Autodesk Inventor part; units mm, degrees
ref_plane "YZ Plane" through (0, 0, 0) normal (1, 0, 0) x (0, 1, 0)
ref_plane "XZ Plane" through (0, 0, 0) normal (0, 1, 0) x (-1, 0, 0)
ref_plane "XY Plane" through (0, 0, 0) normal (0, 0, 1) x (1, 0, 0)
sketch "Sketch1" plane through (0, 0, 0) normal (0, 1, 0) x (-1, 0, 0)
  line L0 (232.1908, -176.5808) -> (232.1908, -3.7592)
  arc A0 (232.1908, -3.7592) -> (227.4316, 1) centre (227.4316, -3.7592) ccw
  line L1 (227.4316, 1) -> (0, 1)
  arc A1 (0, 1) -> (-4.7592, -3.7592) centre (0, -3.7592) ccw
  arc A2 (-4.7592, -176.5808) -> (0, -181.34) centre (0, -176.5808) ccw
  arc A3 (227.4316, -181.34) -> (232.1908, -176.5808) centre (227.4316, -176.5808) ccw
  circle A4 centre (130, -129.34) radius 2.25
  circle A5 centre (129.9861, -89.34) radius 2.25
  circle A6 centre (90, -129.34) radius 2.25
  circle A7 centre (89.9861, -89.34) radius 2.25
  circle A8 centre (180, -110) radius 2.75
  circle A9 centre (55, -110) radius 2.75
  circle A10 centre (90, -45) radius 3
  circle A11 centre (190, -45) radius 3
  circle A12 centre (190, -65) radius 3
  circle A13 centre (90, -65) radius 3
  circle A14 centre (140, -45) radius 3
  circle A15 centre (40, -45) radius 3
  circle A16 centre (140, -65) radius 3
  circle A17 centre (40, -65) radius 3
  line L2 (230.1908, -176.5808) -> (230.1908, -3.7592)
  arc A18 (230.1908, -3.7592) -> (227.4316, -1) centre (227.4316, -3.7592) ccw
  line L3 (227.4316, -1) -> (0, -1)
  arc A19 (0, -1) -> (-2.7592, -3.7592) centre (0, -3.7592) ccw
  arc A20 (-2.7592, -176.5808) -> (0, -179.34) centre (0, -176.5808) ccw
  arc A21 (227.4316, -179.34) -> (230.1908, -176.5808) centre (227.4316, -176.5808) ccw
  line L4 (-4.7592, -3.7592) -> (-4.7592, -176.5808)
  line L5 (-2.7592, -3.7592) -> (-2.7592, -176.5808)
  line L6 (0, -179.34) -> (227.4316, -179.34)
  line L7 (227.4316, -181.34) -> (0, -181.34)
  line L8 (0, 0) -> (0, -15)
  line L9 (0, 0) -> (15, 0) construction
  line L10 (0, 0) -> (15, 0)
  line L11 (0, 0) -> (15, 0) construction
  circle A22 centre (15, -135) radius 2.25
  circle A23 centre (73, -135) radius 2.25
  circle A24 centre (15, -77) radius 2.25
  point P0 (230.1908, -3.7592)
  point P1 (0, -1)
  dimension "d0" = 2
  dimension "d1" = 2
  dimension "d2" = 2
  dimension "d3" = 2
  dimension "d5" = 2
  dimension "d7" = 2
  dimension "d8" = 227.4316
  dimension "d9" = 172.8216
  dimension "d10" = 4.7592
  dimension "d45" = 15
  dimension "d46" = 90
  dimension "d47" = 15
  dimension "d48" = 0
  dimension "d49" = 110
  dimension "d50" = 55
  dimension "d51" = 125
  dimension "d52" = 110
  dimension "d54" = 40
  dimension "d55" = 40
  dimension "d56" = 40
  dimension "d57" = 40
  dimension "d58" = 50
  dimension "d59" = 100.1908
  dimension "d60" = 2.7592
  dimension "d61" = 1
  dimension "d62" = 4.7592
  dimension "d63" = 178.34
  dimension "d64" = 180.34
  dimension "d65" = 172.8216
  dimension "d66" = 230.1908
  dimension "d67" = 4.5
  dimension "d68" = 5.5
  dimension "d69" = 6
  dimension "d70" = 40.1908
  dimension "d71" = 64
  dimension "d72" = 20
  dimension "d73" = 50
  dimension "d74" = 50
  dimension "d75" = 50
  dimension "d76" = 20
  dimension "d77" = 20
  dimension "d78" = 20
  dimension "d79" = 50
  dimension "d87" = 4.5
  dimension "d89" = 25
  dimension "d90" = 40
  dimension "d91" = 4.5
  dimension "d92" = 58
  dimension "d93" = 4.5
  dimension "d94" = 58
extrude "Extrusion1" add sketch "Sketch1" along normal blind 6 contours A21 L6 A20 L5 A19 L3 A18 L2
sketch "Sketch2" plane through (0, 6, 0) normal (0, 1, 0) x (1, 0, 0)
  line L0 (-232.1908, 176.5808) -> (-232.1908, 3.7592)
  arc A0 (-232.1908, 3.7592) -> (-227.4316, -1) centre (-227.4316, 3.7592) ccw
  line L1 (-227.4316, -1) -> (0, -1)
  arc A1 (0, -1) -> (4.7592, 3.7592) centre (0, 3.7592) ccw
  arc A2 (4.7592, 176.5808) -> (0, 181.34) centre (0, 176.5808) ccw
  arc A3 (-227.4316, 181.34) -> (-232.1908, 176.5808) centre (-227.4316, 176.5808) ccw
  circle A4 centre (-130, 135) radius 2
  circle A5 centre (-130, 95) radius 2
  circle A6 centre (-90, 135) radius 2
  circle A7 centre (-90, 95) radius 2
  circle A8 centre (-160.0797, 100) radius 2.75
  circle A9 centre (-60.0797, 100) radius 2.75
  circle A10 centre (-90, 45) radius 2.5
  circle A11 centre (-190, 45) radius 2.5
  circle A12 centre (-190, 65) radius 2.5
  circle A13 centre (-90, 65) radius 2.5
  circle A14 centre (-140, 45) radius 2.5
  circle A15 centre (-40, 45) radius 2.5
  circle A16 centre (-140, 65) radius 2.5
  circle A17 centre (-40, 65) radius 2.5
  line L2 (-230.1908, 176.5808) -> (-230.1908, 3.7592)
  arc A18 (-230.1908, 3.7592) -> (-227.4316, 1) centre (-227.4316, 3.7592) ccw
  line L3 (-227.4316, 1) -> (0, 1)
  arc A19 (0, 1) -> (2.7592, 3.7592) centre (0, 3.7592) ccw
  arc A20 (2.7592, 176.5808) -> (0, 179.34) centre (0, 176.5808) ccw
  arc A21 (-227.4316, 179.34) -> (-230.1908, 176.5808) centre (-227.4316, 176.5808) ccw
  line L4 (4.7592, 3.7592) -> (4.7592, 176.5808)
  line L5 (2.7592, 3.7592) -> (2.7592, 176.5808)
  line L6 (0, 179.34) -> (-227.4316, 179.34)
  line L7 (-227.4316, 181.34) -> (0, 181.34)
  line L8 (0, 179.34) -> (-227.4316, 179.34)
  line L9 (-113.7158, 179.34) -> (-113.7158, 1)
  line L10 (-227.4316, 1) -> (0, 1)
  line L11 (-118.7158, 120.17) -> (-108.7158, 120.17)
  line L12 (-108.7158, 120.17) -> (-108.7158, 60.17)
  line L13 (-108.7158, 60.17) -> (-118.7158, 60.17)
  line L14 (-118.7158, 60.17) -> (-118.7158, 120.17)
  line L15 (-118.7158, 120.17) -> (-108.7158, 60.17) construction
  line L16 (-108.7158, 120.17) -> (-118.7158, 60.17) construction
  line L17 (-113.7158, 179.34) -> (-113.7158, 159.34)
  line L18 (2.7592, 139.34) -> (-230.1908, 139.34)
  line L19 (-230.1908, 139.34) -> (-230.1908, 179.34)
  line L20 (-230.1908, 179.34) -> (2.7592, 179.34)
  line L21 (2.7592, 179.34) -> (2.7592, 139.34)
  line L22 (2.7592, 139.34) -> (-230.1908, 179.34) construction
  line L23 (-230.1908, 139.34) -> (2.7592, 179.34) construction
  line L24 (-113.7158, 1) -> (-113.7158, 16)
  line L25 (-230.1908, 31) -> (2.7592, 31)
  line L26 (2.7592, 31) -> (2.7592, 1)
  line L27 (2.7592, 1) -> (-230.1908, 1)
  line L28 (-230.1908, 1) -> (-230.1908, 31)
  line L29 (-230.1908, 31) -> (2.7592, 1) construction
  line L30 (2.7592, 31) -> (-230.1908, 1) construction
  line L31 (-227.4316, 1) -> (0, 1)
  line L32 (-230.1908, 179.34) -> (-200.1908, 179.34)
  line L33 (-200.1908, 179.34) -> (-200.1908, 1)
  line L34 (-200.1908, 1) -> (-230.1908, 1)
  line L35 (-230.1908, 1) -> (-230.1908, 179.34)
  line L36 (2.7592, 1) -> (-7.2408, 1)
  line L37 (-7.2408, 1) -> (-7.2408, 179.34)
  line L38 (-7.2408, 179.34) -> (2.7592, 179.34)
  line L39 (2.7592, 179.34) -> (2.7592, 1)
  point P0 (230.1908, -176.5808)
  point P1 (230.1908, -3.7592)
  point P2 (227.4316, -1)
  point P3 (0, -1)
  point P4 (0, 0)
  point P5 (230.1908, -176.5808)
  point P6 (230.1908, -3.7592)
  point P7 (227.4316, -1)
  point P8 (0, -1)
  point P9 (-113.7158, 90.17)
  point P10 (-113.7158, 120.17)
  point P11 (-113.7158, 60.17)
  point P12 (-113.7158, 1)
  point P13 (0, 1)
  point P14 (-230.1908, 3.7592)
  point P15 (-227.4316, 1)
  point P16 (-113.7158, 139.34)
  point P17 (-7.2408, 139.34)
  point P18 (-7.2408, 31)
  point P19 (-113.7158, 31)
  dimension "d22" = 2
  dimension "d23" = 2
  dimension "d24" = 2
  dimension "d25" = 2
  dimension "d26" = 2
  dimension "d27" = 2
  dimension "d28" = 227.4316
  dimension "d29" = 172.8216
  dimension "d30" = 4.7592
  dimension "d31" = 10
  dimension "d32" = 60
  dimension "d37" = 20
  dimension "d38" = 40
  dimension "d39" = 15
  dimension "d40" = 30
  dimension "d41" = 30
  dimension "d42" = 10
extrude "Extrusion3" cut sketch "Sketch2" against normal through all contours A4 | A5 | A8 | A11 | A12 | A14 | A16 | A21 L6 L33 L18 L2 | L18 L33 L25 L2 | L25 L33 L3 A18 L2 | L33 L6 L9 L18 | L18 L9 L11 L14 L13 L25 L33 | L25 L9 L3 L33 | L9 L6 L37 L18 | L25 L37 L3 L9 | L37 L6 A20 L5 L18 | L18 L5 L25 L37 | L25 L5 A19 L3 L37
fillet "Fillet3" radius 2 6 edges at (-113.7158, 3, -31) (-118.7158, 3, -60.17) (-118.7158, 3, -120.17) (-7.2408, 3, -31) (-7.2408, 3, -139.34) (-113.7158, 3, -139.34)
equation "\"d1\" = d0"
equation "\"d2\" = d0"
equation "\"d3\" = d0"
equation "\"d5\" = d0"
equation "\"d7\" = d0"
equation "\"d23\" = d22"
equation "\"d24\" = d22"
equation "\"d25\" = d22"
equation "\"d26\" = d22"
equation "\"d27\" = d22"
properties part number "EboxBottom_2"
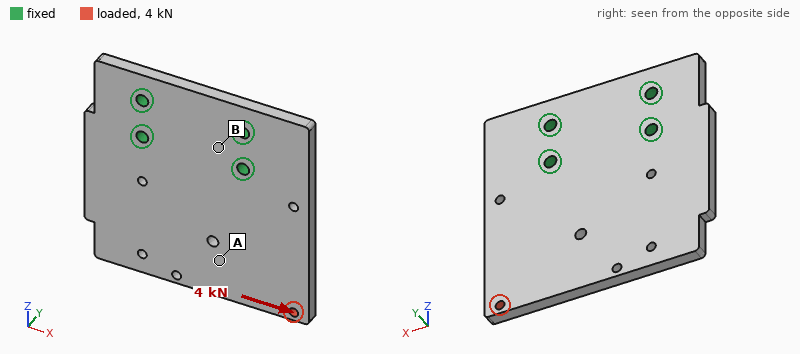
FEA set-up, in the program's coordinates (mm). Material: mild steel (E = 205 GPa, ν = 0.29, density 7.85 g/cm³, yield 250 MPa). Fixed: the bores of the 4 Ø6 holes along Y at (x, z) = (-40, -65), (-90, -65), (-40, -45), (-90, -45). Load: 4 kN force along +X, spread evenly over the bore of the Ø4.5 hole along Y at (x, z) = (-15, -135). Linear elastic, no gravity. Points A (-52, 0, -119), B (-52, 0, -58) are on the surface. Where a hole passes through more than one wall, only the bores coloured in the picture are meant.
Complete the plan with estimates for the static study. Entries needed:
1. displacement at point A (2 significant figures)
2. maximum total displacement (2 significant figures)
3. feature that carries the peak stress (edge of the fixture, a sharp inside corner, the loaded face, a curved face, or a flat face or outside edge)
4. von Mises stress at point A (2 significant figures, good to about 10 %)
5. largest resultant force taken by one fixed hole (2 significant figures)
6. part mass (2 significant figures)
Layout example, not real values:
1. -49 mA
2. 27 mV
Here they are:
1. 12 µm
2. 29 µm
3. the loaded face
4. 23 MPa
5. 4.2 kN
6. 550 g
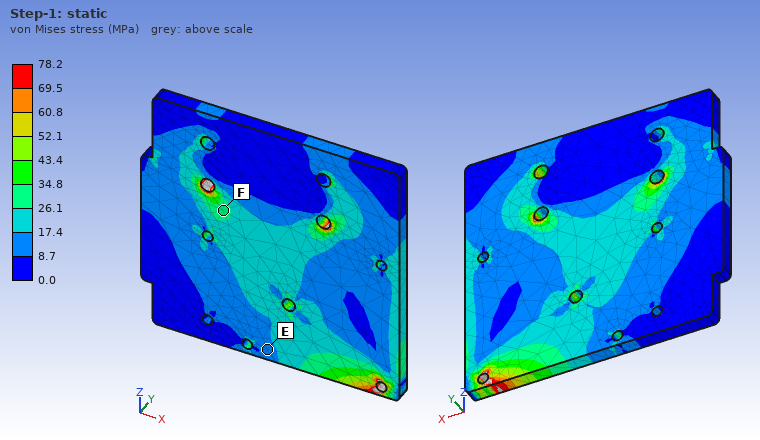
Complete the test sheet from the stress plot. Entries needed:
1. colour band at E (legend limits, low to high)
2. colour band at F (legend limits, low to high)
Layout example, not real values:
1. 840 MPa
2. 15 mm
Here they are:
1. 8.7 to 17.4 MPa
2. 26.1 to 34.8 MPa
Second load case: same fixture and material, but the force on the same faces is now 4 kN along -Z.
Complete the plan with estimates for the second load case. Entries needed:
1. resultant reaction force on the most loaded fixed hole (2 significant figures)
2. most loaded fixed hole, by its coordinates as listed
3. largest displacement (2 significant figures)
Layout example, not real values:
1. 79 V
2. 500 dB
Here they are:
1. 3.7 kN
2. (-40, -65)
3. 18 µm
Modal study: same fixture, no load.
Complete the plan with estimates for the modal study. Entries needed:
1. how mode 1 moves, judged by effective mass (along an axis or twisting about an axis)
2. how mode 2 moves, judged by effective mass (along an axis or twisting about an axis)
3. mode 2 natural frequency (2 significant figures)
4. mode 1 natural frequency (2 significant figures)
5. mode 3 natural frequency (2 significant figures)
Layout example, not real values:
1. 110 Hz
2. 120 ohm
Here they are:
1. along Y
2. twisting about Z
3. 1500 Hz
4. 870 Hz
5. 3300 Hz
